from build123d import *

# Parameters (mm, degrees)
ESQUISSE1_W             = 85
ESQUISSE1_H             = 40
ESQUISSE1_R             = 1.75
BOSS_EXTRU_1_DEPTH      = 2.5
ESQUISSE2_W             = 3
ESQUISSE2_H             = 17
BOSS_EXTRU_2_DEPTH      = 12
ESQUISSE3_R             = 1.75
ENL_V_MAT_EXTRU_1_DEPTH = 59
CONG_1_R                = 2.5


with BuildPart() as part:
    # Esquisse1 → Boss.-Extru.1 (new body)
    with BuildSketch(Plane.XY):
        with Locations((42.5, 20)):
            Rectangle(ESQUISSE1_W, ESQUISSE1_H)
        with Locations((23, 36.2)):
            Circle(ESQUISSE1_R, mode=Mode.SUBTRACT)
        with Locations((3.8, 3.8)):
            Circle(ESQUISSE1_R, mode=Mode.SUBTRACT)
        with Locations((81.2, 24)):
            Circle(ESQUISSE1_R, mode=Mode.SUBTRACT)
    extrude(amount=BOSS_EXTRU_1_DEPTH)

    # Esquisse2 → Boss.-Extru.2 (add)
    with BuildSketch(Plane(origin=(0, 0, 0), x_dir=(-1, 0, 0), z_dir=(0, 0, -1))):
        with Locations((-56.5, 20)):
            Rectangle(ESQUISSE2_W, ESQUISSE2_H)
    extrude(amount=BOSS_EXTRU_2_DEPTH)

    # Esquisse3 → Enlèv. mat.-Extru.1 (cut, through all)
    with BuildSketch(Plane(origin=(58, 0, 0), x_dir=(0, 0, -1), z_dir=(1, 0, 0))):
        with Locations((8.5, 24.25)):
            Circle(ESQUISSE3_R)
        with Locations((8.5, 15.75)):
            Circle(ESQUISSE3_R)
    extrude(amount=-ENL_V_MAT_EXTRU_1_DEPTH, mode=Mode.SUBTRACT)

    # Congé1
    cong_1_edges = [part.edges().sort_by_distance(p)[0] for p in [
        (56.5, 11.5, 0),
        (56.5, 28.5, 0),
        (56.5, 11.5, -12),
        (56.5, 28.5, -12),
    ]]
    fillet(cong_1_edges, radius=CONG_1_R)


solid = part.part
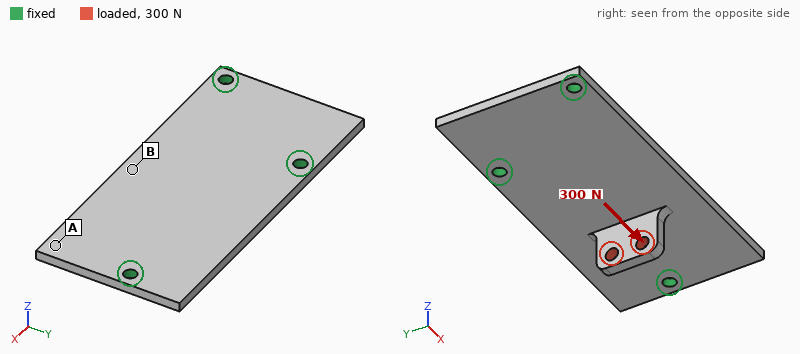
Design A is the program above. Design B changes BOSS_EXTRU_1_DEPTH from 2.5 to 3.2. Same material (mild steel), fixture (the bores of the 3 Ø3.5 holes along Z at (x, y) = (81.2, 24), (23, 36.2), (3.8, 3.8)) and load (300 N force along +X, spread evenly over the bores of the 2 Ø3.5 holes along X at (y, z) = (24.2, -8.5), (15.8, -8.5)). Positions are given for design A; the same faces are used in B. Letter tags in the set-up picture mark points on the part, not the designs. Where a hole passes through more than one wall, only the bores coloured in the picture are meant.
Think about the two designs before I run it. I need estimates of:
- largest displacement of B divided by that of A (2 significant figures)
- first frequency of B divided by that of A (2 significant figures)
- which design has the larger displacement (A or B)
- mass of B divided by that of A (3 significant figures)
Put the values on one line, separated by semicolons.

0.73; 1.3; A; 1.26
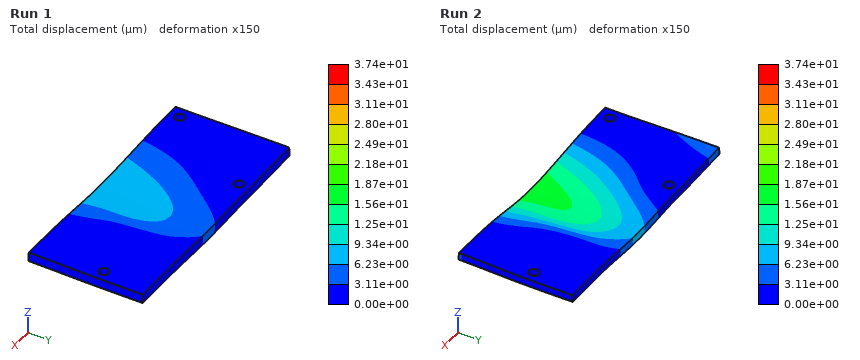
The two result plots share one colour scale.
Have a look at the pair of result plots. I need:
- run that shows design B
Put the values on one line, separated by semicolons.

Run 1
